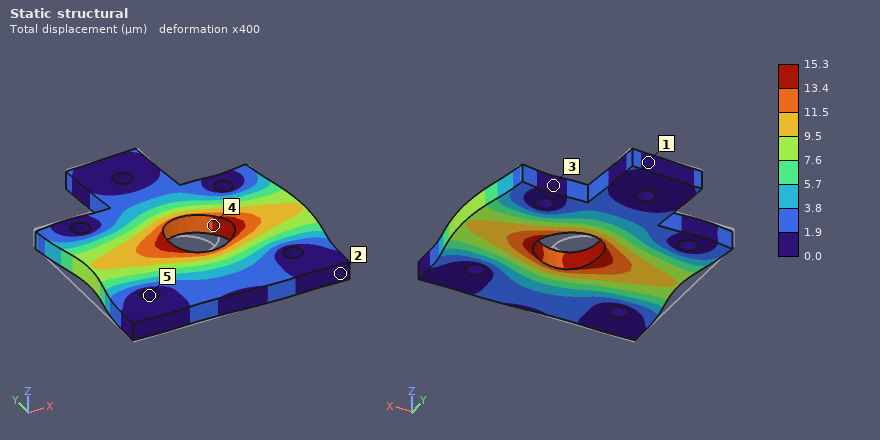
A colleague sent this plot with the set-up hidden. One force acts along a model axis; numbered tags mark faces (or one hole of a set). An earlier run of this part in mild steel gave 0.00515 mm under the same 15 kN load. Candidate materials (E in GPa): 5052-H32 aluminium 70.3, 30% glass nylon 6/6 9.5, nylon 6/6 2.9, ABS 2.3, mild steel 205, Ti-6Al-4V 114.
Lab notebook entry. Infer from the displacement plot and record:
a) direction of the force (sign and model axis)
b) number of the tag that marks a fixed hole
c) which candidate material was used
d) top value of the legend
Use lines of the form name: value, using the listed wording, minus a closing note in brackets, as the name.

direction of the force: +X
number of the tag that marks a fixed hole: 5
which candidate material was used: 5052-H32 aluminium
top value of the legend: 15.3 µm
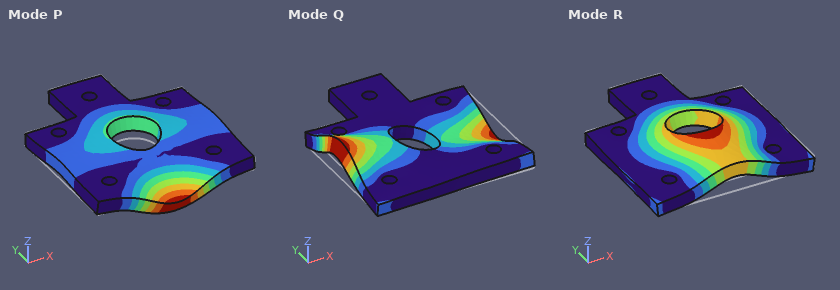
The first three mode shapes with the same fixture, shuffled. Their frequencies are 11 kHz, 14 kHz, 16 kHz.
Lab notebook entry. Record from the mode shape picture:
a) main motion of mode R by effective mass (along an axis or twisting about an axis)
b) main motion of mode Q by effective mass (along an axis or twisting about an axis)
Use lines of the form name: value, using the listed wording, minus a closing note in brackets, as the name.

main motion of mode R by effective mass: along Z
main motion of mode Q by effective mass: twisting about Y
